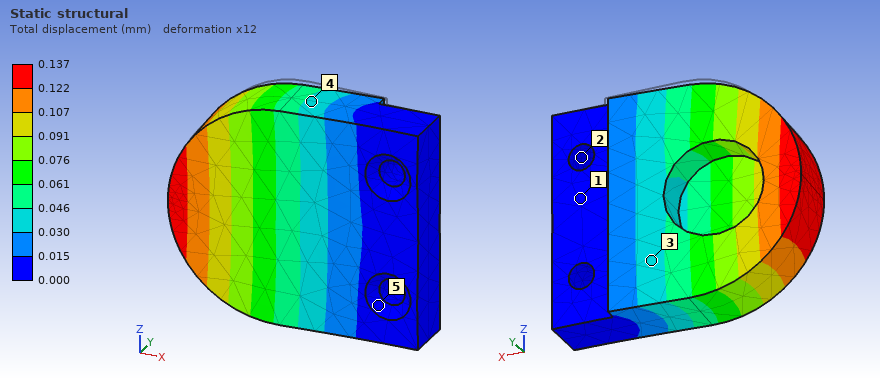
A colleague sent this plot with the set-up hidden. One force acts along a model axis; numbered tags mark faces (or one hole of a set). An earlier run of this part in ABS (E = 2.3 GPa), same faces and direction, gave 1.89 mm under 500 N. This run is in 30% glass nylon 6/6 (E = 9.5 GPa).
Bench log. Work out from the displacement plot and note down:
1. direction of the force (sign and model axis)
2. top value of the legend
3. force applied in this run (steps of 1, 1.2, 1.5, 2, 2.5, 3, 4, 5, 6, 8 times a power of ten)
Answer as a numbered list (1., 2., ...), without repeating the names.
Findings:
1. -Y
2. 0.137 mm
3. 150 N
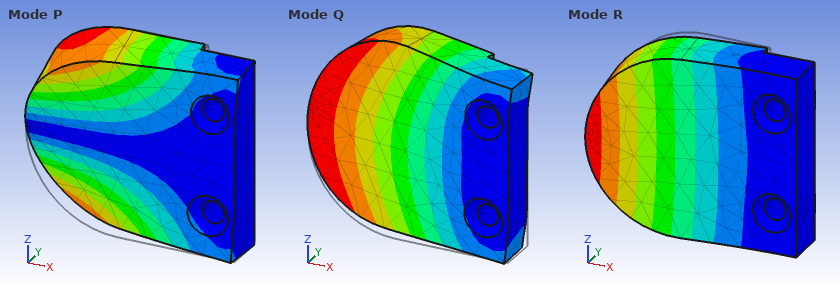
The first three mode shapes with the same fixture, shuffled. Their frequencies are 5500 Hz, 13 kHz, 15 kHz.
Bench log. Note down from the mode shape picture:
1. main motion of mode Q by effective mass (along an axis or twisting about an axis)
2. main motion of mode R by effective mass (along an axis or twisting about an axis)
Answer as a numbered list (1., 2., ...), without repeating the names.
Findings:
1. along Z
2. along Y
